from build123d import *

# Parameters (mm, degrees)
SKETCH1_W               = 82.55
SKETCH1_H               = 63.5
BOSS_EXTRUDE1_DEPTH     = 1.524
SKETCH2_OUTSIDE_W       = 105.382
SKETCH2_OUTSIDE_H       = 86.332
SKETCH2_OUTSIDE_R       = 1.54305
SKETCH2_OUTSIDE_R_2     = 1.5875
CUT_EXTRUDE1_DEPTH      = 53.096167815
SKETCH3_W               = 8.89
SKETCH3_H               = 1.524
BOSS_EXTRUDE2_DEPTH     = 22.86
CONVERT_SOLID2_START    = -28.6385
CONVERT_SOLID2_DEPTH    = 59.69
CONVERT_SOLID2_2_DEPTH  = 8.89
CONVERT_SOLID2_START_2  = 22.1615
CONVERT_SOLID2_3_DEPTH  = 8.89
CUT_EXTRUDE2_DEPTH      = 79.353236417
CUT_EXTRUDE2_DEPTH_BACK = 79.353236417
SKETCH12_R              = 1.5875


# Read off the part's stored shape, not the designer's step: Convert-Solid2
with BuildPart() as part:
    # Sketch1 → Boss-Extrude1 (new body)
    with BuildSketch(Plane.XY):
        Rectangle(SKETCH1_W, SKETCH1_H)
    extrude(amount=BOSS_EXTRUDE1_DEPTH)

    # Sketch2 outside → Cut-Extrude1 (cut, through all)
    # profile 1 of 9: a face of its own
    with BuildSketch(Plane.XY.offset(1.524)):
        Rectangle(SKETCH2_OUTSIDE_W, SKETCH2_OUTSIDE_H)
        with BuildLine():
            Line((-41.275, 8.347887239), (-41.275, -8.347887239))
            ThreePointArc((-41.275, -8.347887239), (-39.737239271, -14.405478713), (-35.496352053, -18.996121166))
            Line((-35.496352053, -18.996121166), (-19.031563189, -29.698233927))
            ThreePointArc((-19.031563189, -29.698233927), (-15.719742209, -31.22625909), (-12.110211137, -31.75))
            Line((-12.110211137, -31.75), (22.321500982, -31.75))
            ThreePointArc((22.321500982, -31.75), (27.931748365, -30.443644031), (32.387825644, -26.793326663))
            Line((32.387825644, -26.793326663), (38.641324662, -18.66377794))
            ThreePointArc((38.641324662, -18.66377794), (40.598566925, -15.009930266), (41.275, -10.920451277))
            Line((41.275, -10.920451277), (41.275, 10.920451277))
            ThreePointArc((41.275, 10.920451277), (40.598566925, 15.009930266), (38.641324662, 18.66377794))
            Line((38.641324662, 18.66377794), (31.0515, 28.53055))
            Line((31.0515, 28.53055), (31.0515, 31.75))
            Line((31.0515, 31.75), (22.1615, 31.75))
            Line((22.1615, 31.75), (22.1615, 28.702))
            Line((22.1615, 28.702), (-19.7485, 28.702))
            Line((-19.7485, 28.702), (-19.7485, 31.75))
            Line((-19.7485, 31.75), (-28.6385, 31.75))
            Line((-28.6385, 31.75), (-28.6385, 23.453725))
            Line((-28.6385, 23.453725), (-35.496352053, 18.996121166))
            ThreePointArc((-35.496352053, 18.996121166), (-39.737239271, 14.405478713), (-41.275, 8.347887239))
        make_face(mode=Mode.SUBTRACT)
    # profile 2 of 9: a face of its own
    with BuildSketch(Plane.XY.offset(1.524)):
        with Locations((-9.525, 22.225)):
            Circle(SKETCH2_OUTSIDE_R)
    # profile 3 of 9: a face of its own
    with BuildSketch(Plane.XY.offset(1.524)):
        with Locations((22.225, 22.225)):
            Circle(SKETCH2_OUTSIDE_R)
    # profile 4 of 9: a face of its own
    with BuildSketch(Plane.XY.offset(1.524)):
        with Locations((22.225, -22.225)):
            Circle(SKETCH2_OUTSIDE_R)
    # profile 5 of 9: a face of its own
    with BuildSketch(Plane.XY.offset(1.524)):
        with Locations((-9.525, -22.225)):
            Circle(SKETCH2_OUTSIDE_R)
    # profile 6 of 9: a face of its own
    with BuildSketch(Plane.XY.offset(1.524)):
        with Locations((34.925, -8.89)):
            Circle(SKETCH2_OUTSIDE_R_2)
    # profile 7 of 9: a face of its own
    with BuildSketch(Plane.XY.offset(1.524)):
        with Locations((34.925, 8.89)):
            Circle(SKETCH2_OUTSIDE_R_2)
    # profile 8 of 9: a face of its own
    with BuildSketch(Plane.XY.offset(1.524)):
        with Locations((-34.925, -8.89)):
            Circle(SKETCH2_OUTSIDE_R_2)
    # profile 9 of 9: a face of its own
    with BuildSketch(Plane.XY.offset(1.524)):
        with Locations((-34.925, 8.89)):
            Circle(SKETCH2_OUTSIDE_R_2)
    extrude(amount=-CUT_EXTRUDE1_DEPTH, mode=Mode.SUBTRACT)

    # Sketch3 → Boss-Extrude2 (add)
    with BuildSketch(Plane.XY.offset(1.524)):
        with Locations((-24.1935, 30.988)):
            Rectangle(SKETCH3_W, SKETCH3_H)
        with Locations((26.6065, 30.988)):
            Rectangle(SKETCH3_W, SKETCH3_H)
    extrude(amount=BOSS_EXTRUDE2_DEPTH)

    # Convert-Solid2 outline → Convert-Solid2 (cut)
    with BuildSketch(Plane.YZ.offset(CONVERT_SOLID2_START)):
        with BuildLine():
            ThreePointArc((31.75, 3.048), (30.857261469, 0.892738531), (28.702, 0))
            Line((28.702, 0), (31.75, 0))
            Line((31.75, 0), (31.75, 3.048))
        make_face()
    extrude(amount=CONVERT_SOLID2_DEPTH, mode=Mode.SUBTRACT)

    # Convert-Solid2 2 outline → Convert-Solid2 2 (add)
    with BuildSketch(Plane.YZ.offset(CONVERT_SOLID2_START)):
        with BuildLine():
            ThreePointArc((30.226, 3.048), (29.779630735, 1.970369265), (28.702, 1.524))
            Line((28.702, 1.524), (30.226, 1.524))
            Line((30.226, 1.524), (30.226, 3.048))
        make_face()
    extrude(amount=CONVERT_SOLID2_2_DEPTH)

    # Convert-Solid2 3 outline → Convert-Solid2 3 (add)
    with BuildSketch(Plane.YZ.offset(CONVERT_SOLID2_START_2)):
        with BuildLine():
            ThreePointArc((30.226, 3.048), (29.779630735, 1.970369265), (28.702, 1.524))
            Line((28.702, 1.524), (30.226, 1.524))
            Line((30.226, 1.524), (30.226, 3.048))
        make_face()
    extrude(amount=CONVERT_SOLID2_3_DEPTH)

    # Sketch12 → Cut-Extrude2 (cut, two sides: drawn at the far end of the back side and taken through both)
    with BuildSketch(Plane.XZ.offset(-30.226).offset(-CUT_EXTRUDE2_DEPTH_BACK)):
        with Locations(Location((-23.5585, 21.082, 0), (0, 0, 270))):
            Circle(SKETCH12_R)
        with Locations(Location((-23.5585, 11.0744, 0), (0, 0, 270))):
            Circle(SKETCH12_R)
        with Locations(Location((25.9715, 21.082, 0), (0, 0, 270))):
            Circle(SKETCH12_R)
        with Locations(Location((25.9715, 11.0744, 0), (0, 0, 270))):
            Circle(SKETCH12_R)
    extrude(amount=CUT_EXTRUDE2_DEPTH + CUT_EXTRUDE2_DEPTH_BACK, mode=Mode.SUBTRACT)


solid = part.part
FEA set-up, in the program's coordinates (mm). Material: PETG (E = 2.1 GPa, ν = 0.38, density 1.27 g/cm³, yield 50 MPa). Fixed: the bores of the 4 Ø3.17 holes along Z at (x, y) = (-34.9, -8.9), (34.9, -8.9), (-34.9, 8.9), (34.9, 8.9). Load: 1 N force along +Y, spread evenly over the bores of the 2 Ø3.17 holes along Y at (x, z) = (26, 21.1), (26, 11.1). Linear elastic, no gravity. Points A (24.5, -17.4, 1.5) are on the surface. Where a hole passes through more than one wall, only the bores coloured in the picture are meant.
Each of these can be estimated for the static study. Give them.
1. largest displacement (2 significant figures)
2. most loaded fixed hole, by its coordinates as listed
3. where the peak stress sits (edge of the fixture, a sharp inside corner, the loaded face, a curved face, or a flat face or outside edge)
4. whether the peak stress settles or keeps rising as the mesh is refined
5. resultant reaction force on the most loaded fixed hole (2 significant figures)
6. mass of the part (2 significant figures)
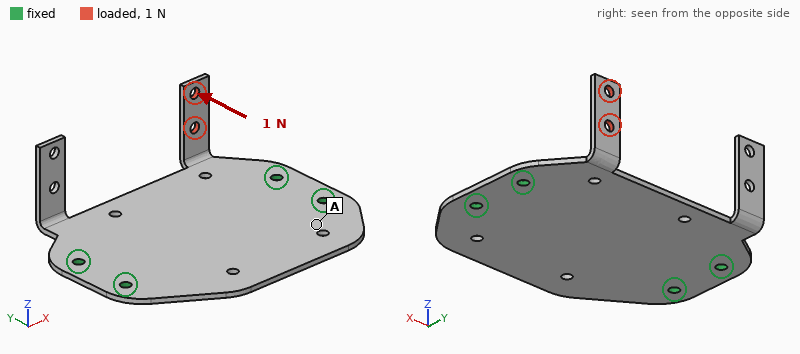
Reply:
1.1 mm
(34.9, 8.9)
a sharp inside corner
keeps rising
0.70 N
9.3 g
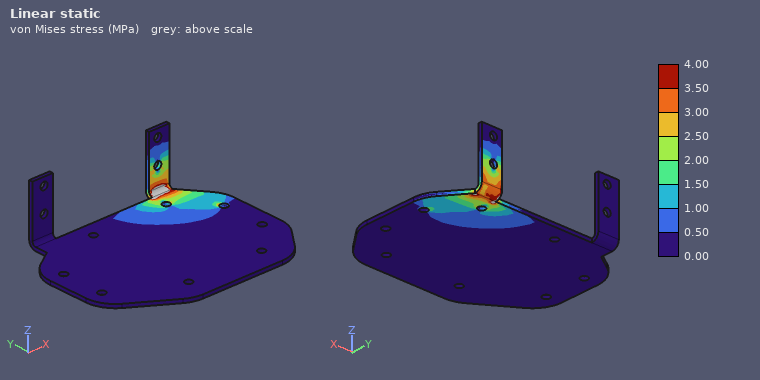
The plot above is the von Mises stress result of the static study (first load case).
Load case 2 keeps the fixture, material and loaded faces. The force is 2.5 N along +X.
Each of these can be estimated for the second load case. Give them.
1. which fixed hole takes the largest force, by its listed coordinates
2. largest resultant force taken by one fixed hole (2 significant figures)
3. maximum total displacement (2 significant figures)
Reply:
(34.9, 8.9)
1.7 N
1.1 mm
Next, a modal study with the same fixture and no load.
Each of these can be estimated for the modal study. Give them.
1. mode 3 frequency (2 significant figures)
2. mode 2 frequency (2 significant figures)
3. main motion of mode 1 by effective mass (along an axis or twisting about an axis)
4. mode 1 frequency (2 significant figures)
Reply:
330 Hz
330 Hz
along Z
270 Hz
